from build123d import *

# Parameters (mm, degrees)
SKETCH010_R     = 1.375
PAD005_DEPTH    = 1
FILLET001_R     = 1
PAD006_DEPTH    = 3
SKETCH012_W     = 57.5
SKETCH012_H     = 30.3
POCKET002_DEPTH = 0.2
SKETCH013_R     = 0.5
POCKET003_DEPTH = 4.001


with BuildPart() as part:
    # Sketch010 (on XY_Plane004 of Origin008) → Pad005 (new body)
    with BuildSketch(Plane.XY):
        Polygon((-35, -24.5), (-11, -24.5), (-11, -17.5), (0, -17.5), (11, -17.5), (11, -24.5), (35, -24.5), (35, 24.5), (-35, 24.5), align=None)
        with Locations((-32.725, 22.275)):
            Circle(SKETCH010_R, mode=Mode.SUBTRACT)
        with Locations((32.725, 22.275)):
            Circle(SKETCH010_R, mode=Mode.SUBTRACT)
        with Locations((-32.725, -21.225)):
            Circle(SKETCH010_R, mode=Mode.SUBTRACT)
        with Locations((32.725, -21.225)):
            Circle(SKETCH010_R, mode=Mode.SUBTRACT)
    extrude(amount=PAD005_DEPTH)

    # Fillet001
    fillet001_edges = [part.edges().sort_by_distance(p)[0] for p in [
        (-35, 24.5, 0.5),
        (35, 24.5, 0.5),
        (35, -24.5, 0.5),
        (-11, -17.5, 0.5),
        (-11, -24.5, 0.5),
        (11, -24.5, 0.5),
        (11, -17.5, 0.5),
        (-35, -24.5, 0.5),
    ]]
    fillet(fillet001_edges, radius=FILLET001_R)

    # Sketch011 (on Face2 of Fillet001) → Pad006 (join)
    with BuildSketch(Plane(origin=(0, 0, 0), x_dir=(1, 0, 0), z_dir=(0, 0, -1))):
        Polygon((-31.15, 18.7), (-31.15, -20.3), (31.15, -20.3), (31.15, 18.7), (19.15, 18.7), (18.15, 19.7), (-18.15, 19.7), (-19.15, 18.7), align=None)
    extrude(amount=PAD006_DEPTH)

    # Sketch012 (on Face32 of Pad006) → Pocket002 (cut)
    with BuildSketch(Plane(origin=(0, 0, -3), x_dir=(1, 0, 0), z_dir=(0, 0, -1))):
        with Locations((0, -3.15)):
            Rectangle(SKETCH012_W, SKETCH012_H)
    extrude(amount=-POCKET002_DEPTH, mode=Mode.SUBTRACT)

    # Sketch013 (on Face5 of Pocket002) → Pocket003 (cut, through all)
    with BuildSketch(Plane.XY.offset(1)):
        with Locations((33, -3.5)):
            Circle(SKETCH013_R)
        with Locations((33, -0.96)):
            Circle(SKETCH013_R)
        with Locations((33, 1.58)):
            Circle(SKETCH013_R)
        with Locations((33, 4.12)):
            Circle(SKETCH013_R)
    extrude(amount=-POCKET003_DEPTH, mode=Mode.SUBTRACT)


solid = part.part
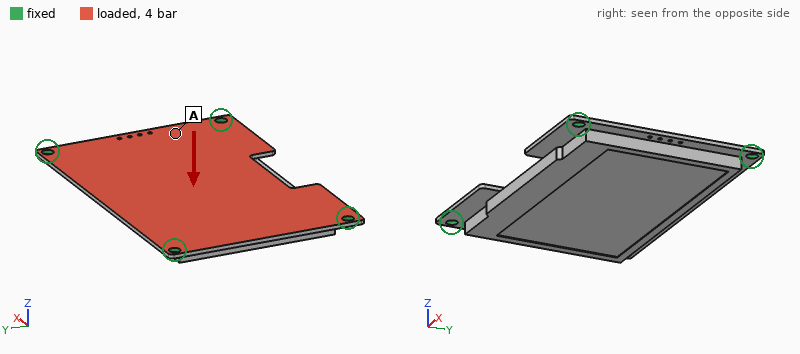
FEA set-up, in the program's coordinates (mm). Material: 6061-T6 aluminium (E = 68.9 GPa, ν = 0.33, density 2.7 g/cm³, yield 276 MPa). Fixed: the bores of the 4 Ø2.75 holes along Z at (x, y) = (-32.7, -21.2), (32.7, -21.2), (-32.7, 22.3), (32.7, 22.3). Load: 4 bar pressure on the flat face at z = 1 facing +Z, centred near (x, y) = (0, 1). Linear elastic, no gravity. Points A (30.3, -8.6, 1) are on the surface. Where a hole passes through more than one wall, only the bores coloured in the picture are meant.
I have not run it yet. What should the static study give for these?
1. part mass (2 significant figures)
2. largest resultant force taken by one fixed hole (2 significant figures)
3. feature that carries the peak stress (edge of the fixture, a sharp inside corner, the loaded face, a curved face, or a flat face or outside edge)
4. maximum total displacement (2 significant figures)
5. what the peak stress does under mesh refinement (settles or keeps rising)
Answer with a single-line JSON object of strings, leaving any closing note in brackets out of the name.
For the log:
{"part mass": "28 g", "largest resultant force taken by one fixed hole": "900 N", "feature that carries the peak stress": "edge of the fixture", "maximum total displacement": "0.25 mm", "what the peak stress does under mesh refinement": "keeps rising"}
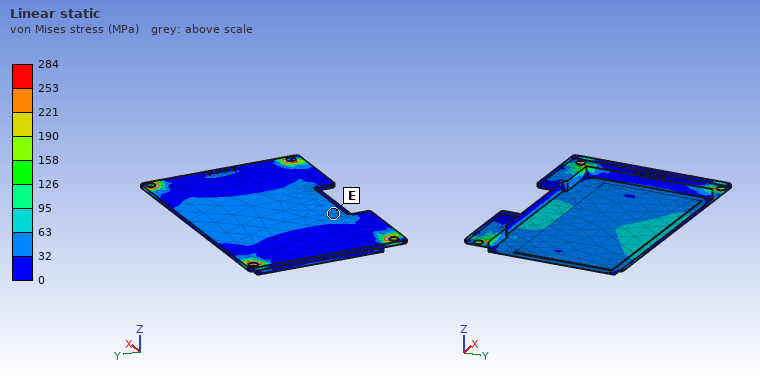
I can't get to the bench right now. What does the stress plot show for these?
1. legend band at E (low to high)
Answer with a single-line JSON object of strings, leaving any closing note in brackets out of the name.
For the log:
{"legend band at E": "32 to 63 MPa"}
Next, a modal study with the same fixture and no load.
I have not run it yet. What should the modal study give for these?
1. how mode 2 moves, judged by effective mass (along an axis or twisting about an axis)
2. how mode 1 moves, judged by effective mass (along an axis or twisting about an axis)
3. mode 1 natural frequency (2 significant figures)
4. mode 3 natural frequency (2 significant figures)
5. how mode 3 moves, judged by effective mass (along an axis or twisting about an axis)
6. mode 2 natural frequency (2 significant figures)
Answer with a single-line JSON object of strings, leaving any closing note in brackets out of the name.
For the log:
{"how mode 2 moves, judged by effective mass": "twisting about X", "how mode 1 moves, judged by effective mass": "along Z", "mode 1 natural frequency": "2500 Hz", "mode 3 natural frequency": "5800 Hz", "how mode 3 moves, judged by effective mass": "twisting about Y", "mode 2 natural frequency": "4700 Hz"}
